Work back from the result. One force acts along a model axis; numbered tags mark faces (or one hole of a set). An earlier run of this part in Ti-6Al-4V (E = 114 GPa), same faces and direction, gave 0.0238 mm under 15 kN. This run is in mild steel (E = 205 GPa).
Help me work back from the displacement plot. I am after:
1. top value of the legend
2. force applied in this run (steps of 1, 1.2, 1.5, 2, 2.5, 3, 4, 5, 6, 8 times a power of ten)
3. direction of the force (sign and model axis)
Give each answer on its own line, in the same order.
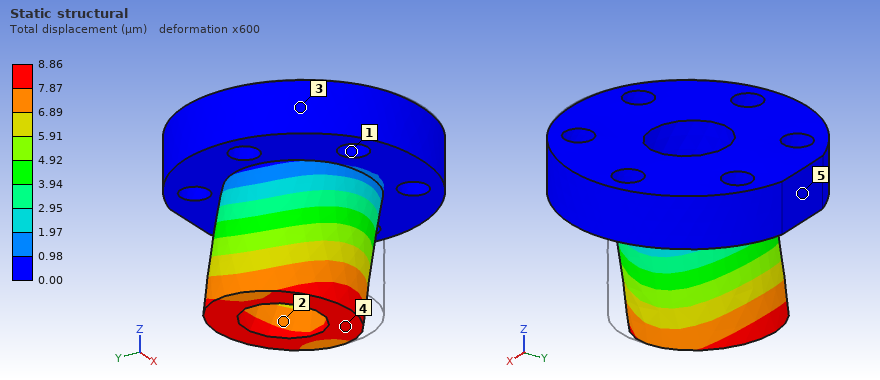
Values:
8.86 µm
10 kN
+Y
